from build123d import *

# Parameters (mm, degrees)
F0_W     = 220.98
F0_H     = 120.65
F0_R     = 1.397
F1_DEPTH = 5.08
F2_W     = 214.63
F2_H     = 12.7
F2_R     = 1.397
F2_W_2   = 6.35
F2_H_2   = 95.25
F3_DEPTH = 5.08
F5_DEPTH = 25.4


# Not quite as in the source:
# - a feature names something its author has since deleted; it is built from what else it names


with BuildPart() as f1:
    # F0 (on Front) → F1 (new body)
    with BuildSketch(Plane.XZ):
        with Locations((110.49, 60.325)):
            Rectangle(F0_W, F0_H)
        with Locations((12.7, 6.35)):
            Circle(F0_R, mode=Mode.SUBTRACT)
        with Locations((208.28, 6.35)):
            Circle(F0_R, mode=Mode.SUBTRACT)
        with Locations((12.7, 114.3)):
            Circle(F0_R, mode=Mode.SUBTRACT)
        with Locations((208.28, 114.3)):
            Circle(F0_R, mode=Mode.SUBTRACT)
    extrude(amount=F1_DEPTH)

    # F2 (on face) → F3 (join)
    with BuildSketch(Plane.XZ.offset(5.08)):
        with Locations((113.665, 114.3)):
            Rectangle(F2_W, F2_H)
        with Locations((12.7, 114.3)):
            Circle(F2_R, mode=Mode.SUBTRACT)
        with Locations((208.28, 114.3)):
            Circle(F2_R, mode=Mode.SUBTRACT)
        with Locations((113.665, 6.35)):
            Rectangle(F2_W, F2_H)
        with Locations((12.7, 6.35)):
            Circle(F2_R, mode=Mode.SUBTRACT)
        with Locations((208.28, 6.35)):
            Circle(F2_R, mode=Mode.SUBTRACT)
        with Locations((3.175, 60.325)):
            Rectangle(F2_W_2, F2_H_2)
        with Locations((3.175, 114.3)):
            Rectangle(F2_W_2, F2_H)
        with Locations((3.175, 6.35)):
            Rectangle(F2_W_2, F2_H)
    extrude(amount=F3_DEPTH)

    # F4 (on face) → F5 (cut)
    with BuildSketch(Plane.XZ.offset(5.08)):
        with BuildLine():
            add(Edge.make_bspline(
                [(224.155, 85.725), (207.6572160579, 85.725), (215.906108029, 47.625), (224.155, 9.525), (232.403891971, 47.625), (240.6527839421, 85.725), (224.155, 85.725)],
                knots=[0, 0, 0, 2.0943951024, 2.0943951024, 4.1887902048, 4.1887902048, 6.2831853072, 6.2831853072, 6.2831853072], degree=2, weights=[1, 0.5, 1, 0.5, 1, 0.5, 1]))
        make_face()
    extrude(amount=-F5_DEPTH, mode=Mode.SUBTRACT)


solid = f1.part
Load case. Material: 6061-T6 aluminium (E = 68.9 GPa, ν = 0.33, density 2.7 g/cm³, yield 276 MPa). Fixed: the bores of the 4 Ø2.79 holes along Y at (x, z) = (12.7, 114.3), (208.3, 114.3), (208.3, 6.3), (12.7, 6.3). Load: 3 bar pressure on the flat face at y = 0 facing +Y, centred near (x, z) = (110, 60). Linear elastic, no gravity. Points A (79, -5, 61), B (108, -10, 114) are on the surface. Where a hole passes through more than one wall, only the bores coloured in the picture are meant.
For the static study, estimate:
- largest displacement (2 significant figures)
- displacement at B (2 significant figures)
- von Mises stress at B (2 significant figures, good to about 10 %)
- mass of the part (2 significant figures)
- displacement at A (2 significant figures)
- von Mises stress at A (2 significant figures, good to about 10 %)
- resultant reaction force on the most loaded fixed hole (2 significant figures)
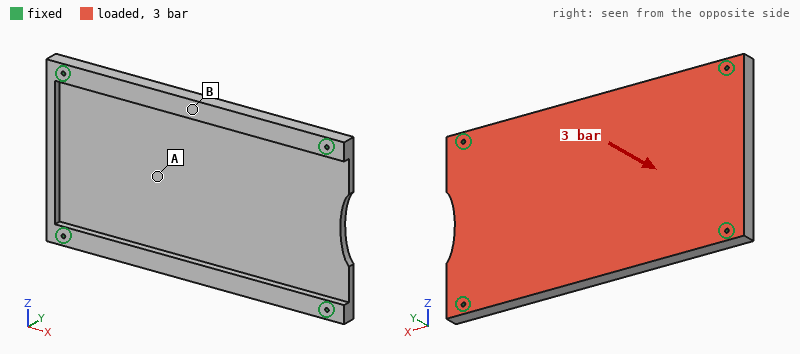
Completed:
0.84 mm
0.61 mm
94 MPa
450 g
0.73 mm
45 MPa
3.0 kN
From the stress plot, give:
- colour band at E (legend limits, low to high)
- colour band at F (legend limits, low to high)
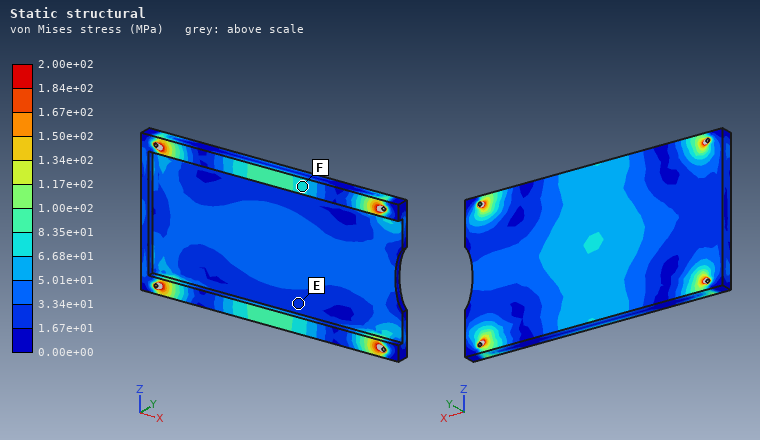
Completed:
1.67e+01 to 3.34e+01 MPa
6.68e+01 to 8.35e+01 MPa
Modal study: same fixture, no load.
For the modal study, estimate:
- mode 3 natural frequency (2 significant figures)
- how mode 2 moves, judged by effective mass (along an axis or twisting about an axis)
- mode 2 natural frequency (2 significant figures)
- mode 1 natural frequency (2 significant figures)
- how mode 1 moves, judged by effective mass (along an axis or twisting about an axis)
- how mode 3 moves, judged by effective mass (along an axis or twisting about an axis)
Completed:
2100 Hz
twisting about X
1400 Hz
910 Hz
along Y
twisting about Z
